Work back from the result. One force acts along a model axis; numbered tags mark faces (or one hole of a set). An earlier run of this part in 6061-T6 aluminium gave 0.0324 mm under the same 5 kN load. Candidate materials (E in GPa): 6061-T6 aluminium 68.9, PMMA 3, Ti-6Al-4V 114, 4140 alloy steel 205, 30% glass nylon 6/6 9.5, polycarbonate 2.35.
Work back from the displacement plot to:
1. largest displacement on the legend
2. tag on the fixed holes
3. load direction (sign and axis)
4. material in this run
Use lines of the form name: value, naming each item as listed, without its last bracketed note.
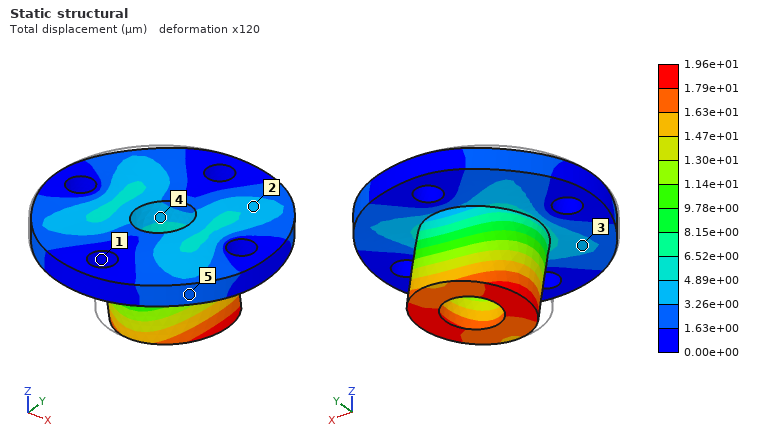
largest displacement on the legend: 1.96e+01 µm
tag on the fixed holes: 1
load direction: +X
material in this run: Ti-6Al-4V
